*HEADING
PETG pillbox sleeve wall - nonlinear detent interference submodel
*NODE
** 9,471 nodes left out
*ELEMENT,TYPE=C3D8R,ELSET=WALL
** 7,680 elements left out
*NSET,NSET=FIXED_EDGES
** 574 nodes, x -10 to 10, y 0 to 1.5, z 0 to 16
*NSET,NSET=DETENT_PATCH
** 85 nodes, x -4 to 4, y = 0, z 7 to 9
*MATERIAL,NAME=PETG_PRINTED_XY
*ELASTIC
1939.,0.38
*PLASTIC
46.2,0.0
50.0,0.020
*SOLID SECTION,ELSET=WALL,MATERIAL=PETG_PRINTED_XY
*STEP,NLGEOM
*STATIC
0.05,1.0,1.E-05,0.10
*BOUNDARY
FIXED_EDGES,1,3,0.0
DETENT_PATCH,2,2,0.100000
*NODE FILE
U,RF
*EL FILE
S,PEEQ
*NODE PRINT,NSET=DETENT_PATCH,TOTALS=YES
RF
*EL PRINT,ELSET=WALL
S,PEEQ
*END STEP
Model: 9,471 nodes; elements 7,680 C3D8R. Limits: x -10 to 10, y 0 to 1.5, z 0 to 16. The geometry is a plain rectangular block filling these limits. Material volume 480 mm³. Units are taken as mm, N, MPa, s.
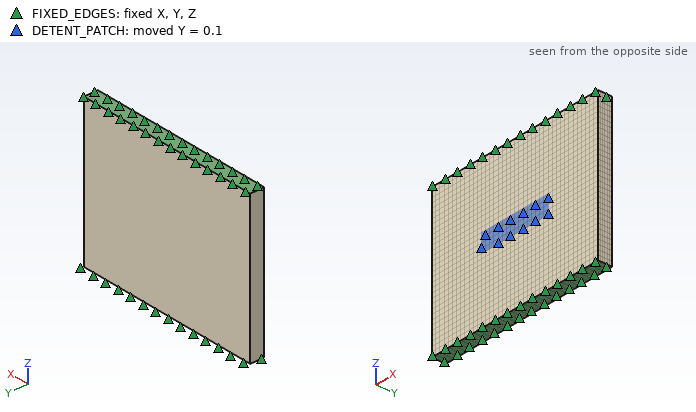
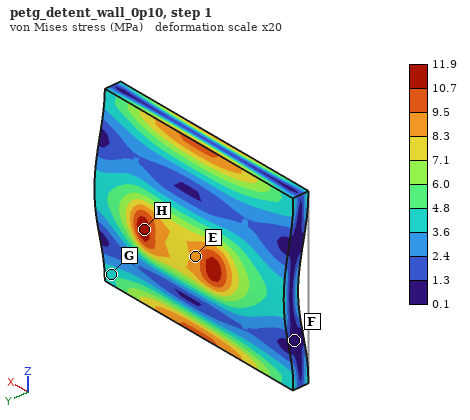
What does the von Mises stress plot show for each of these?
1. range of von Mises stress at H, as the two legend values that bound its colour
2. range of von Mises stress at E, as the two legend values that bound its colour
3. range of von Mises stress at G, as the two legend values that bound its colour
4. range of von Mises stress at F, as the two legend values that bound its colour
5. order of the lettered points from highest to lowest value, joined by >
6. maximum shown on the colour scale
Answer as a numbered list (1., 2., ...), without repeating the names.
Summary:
1. 10.7 to 11.9 MPa
2. 8.3 to 9.5 MPa
3. 3.6 to 4.8 MPa
4. 0.1 to 1.3 MPa
5. H > E > G > F
6. 11.9 MPa
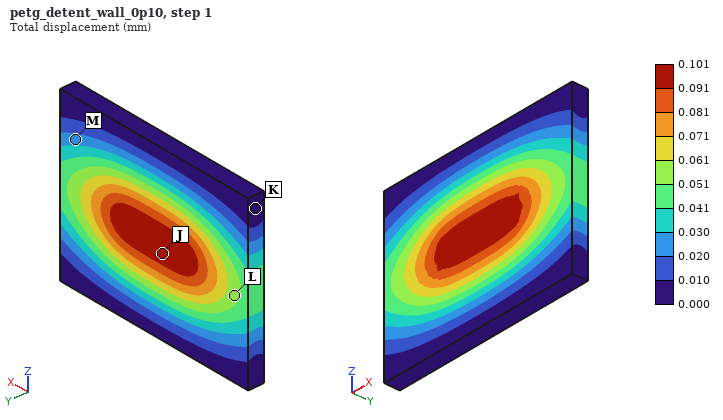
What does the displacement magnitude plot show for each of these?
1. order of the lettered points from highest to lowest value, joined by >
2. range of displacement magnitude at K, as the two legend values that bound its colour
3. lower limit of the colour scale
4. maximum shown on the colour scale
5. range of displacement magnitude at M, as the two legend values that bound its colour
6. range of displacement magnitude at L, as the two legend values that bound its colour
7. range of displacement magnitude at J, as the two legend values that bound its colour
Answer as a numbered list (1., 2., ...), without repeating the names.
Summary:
1. J > L > M > K
2. 0.000 to 0.010 mm
3. 0.000 mm
4. 0.101 mm
5. 0.020 to 0.030 mm
6. 0.051 to 0.061 mm
7. 0.091 to 0.101 mm
